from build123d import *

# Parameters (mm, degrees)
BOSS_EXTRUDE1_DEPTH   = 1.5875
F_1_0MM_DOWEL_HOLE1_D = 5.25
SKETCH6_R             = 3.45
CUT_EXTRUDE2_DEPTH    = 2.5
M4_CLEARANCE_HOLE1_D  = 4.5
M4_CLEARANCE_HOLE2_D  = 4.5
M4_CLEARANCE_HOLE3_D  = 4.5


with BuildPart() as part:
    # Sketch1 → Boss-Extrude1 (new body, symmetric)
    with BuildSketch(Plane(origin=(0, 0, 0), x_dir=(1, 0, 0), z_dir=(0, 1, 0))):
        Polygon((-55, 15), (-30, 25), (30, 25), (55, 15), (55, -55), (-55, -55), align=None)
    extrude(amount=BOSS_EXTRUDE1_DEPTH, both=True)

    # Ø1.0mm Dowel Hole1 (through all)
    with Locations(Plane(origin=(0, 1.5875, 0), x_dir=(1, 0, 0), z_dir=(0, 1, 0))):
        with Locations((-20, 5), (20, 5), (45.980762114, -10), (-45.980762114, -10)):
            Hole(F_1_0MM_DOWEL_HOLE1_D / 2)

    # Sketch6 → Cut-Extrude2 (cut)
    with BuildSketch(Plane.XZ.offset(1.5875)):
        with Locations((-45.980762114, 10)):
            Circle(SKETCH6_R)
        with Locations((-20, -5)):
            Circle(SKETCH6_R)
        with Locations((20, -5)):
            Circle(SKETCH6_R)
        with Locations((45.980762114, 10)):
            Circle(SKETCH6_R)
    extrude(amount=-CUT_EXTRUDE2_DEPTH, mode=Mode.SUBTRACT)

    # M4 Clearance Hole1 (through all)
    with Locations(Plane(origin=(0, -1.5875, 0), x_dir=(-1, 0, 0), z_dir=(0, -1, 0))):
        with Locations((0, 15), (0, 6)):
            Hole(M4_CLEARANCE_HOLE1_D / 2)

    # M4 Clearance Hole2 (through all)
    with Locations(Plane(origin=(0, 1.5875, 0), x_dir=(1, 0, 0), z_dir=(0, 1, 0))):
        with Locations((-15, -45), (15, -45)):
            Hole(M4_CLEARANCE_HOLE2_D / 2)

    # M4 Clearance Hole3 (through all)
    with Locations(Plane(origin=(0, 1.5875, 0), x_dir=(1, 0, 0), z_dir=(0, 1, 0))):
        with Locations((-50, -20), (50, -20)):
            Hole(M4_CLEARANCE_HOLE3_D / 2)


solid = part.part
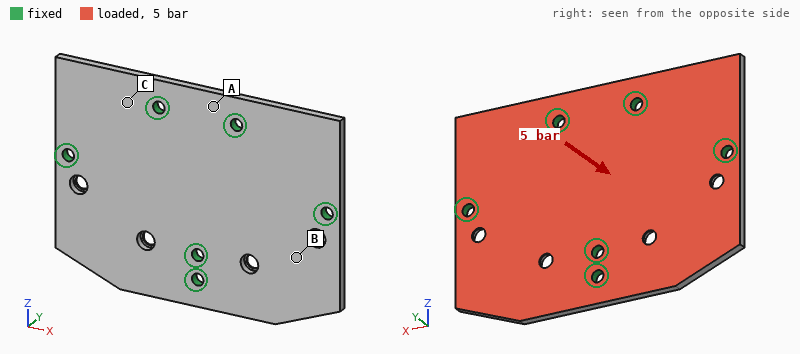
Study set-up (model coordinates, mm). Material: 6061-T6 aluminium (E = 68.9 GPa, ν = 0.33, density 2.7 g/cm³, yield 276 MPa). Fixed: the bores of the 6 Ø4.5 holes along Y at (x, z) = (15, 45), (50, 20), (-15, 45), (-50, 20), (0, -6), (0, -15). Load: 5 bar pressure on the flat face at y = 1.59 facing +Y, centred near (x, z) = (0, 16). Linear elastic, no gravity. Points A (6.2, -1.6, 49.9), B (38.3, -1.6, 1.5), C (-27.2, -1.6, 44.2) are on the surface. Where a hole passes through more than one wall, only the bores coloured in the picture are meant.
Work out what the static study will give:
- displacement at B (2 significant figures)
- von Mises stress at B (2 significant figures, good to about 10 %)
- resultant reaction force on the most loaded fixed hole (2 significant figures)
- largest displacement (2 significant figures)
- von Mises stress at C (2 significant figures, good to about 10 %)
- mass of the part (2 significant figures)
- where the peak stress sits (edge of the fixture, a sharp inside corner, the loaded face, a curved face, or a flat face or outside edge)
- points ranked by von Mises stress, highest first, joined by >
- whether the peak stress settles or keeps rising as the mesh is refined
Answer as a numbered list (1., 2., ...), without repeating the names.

1. 0.15 mm
2. 57 MPa
3. 810 N
4. 0.39 mm
5. 31 MPa
6. 71 g
7. edge of the fixture
8. B > C > A
9. keeps rising
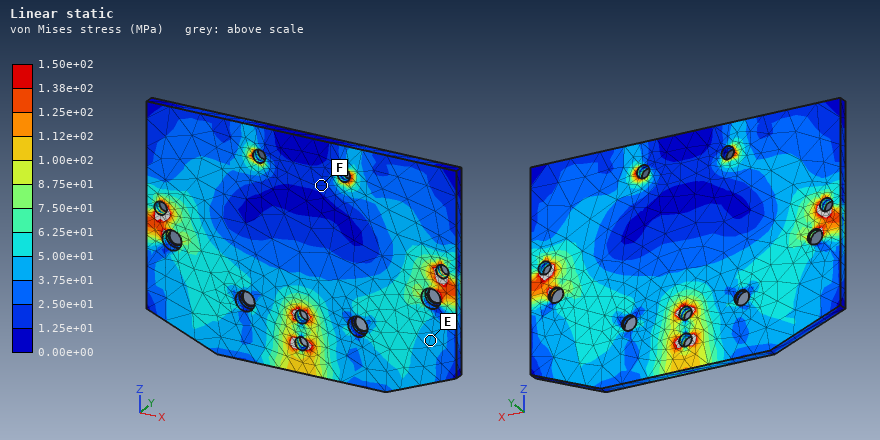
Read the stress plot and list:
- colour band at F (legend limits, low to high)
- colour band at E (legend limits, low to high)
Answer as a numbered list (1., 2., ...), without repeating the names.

1. 1.25e+01 to 2.50e+01 MPa
2. 3.75e+01 to 5.00e+01 MPa
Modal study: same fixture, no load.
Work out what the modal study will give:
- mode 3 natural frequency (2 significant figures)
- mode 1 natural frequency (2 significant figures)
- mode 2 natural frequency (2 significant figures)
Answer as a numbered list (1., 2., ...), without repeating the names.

1. 3800 Hz
2. 2500 Hz
3. 2600 Hz
